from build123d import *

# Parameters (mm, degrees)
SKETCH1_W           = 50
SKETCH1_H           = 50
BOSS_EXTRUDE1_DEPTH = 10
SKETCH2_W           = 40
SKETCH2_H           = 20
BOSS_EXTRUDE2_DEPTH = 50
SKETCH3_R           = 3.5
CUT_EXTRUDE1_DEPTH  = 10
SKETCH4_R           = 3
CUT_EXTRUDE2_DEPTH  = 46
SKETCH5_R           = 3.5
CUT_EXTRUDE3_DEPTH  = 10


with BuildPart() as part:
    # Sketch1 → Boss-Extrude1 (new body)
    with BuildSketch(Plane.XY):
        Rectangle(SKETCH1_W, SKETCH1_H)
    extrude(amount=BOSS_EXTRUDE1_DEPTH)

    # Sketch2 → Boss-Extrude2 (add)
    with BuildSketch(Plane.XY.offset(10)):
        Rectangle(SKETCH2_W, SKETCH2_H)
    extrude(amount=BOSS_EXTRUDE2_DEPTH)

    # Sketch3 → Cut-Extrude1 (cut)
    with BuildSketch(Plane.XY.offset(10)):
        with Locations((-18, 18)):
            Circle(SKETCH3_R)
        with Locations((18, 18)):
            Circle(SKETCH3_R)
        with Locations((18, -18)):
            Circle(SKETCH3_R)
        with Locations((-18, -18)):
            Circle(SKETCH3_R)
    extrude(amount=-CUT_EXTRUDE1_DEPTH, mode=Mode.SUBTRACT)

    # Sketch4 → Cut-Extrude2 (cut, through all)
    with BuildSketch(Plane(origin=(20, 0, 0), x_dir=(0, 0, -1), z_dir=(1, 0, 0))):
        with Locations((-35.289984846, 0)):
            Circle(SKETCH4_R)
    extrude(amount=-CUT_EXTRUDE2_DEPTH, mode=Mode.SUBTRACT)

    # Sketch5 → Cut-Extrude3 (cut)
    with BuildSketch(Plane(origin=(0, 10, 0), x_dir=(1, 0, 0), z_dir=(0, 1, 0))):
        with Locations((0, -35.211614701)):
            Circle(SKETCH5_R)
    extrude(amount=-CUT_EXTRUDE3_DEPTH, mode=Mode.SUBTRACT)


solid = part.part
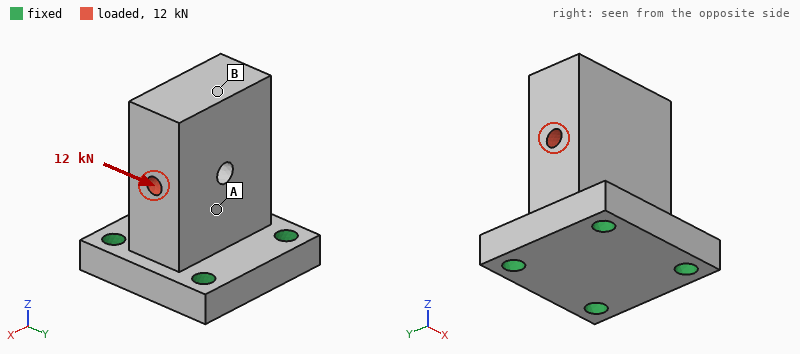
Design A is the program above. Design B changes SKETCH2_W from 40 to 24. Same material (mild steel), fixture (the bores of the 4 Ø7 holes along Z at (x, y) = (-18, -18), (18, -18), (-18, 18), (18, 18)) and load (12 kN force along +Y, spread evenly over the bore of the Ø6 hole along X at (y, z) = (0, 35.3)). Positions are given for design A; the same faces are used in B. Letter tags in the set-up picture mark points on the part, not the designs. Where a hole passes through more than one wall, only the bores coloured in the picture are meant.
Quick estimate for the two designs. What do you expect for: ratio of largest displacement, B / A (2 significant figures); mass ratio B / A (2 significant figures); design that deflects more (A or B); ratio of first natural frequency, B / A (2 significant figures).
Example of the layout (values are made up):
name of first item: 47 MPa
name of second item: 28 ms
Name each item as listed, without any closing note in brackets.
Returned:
ratio of largest displacement, B / A: 1.7
mass ratio B / A: 0.75
design that deflects more: B
ratio of first natural frequency, B / A: 0.99
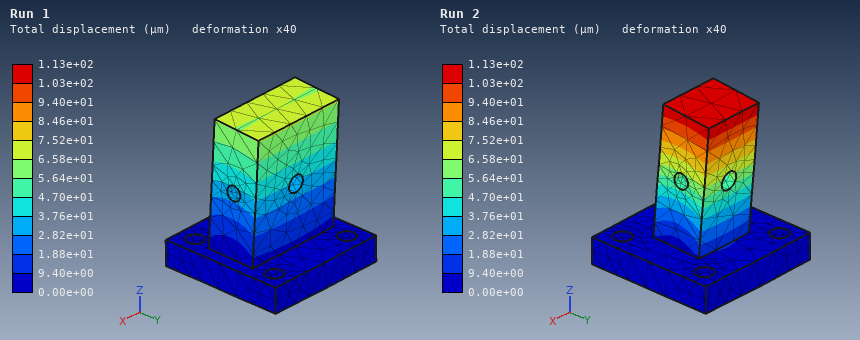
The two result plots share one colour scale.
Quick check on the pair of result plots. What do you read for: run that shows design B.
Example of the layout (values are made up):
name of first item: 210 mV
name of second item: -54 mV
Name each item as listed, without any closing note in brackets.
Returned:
run that shows design B: Run 2
